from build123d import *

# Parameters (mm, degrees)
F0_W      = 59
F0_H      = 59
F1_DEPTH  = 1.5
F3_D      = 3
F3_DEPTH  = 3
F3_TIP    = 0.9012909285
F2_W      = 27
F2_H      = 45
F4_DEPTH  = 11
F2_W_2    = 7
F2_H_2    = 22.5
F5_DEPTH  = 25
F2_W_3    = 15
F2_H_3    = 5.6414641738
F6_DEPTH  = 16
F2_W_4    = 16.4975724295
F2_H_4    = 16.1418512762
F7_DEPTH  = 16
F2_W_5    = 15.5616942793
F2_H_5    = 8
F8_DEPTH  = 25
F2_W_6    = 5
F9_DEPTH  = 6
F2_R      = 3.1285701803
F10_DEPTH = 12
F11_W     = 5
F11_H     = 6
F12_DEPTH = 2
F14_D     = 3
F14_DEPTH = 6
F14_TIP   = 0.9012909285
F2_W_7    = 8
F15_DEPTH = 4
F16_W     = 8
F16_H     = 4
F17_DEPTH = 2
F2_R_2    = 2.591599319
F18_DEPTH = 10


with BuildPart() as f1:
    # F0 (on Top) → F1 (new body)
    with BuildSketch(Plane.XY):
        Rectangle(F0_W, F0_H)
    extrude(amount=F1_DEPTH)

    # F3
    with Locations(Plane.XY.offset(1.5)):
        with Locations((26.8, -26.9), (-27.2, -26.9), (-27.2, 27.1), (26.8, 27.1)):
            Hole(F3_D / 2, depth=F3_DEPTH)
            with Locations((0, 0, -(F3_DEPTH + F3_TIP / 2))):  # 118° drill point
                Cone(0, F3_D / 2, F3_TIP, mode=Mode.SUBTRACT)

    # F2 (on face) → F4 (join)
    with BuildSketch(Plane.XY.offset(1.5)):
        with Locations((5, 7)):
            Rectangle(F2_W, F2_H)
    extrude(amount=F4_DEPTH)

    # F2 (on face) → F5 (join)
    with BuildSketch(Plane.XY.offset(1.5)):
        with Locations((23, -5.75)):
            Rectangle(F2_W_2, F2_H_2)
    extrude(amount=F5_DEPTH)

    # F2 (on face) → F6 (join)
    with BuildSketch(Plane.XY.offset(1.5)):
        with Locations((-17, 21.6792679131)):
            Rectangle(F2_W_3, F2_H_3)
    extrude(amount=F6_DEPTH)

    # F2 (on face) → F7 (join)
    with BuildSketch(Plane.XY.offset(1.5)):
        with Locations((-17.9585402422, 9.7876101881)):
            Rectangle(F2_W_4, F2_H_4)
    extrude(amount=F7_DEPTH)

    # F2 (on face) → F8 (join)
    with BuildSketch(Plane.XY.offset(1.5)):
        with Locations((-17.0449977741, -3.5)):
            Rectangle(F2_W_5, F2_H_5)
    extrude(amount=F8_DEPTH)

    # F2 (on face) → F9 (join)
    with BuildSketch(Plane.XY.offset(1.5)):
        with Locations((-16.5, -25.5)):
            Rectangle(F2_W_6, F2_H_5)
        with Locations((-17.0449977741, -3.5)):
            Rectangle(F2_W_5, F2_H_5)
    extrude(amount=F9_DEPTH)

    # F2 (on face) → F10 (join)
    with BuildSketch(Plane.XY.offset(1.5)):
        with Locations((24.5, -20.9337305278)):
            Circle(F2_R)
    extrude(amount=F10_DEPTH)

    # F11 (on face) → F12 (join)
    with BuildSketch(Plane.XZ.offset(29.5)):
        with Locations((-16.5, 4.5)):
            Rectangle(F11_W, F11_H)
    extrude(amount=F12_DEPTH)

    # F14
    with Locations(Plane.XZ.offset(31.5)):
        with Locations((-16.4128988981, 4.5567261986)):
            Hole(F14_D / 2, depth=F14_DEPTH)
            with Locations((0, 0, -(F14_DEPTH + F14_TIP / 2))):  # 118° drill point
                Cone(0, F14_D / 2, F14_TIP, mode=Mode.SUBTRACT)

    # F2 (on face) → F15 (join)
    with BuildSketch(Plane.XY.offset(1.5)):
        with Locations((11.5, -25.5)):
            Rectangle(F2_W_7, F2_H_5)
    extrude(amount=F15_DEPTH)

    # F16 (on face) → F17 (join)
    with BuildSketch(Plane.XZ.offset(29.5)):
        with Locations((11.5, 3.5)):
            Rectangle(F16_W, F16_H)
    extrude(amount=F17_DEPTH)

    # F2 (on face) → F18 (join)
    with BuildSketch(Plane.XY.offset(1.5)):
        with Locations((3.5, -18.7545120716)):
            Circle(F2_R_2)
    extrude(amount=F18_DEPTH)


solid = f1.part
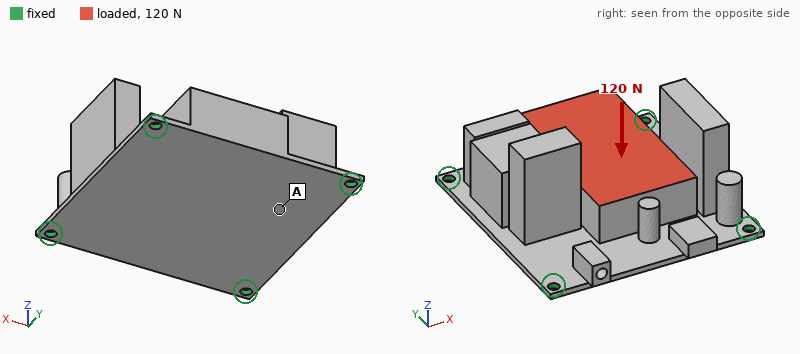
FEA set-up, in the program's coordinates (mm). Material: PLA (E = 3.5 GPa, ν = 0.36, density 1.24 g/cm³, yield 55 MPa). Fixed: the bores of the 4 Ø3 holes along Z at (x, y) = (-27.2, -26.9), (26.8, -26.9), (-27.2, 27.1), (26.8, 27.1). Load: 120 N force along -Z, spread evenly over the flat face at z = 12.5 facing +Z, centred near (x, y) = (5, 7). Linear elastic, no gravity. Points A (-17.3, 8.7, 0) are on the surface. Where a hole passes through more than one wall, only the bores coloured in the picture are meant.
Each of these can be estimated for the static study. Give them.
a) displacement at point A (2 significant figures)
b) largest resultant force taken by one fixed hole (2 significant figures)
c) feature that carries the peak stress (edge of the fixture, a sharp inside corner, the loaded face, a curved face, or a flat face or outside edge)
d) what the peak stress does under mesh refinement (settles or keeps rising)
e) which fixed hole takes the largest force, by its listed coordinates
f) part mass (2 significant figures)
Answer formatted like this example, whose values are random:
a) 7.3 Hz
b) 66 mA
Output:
a) 0.31 mm
b) 52 N
c) edge of the fixture
d) keeps rising
e) (-27.2, 27.1)
f) 40 g
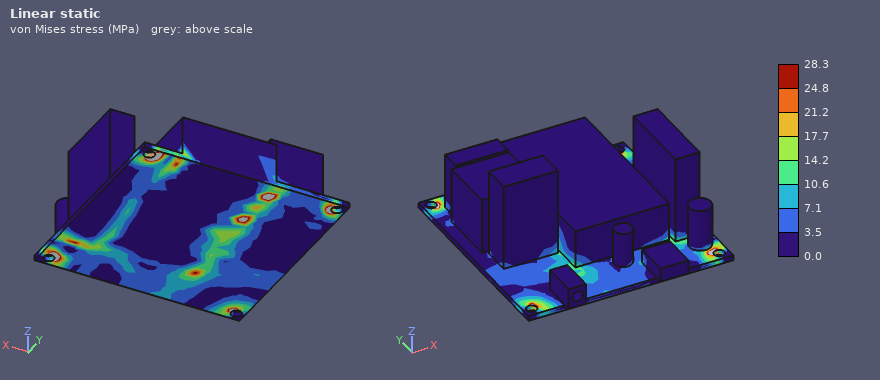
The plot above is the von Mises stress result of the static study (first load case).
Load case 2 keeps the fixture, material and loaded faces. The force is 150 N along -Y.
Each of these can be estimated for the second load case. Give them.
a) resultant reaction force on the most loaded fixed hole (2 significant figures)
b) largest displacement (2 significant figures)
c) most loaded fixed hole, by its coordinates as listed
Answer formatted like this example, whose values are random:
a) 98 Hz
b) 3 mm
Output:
a) 66 N
b) 0.34 mm
c) (26.8, -26.9)
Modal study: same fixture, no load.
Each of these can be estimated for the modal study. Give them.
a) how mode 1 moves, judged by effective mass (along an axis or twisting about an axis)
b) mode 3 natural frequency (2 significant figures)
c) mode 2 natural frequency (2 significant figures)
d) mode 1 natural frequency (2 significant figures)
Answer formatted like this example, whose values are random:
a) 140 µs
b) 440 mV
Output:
a) along Z
b) 730 Hz
c) 680 Hz
d) 430 Hz
